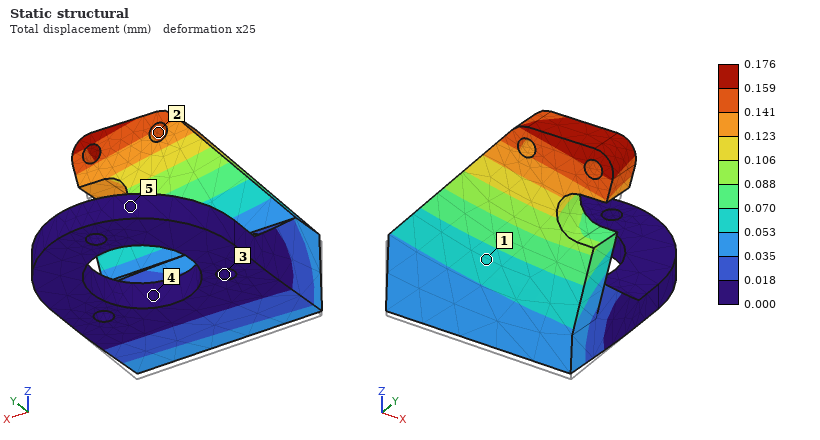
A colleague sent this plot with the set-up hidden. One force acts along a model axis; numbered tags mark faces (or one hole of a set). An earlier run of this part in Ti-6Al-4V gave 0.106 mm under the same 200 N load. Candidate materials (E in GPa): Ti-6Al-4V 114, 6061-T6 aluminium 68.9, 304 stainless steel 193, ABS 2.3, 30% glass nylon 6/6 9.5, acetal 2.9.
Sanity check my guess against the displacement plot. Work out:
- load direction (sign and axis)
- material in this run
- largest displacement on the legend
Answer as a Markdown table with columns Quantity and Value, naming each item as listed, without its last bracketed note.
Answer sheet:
| Quantity | Value |
|---|---|
| load direction | +Y |
| material in this run | 6061-T6 aluminium |
| largest displacement on the legend | 0.176 mm |
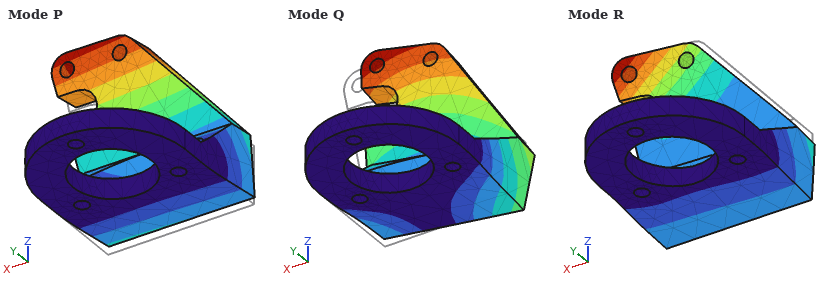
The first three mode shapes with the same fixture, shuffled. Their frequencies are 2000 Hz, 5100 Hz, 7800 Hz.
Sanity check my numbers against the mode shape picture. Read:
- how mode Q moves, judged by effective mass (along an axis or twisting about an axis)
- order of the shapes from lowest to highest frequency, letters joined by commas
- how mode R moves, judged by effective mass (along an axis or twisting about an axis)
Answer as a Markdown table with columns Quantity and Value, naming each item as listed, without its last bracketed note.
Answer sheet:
| Quantity | Value |
|---|---|
| how mode Q moves, judged by effective mass | along X |
| order of the shapes from lowest to highest frequency, letters joined by commas | P, Q, R |
| how mode R moves, judged by effective mass | along Z |
